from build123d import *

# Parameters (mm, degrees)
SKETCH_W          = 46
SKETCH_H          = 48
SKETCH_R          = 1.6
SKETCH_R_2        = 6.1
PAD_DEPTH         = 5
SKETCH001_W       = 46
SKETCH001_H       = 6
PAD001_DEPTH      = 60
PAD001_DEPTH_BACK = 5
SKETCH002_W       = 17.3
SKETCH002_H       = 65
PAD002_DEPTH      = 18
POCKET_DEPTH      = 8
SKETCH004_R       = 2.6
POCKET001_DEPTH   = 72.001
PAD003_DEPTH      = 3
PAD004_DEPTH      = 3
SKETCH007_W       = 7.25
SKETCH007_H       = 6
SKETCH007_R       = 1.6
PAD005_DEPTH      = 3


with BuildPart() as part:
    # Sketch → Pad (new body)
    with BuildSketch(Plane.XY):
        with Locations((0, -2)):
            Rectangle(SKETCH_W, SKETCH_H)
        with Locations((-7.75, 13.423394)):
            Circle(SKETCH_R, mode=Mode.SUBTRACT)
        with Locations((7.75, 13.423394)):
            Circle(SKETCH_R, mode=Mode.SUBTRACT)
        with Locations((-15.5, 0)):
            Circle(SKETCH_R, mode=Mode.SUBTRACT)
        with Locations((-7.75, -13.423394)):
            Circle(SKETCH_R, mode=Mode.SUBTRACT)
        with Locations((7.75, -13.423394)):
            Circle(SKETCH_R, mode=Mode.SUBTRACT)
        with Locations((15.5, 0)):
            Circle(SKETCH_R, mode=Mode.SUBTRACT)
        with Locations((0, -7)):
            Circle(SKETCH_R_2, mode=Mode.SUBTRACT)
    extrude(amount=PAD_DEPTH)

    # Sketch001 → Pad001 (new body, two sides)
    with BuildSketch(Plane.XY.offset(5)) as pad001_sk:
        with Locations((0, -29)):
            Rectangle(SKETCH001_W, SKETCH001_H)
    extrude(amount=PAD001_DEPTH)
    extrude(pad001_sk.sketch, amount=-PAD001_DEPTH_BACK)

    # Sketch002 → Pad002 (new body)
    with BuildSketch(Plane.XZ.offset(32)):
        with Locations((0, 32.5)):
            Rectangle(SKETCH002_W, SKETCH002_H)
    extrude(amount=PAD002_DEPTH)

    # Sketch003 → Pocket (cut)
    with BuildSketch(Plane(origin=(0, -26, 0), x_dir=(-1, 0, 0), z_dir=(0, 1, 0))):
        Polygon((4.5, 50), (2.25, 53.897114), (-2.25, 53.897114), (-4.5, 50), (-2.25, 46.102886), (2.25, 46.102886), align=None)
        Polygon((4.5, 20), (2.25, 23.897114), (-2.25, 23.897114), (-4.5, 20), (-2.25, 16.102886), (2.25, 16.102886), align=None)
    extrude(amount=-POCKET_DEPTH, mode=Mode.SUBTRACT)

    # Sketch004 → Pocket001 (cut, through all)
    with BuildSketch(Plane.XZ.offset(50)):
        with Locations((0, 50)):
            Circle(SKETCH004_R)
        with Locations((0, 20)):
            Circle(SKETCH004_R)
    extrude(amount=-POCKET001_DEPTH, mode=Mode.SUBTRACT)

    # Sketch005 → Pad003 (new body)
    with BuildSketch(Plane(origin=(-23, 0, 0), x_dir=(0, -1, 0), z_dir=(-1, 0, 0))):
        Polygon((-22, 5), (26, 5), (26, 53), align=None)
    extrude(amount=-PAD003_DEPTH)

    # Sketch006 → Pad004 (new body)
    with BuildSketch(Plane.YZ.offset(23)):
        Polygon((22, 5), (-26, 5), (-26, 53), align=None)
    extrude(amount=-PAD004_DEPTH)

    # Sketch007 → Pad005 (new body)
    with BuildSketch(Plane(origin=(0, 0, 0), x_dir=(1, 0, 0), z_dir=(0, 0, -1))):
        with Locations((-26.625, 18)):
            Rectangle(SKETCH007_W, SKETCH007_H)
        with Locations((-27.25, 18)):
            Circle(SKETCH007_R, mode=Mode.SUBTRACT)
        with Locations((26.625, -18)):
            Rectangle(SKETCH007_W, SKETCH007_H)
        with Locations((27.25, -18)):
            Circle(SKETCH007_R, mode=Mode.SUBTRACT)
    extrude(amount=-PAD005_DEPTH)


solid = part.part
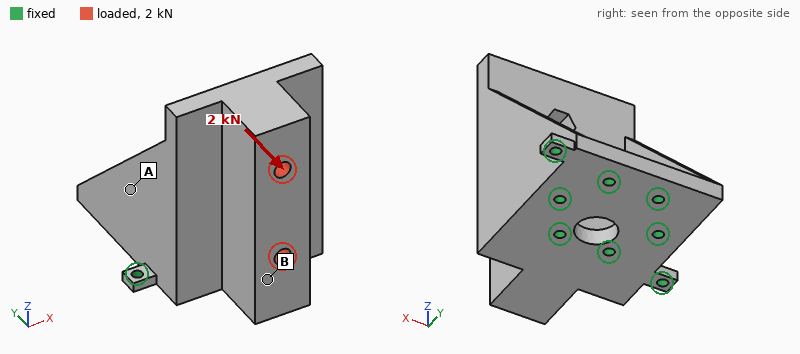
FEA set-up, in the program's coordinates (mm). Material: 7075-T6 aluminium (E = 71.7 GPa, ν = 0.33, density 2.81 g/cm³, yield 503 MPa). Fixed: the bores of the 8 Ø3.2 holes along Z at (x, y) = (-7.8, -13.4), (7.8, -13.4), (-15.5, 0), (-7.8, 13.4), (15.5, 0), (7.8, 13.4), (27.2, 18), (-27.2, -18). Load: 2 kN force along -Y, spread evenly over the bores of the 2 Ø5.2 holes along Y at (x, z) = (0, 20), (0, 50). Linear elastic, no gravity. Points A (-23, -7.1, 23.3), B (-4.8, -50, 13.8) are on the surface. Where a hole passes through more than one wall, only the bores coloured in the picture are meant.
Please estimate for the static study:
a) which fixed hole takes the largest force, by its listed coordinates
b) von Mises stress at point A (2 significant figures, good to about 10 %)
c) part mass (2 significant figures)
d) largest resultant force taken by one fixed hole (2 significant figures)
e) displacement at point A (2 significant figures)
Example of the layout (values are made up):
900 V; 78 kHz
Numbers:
(-15.5, 0); 19 MPa; 150 g; 1.2 kN; 0.042 mm
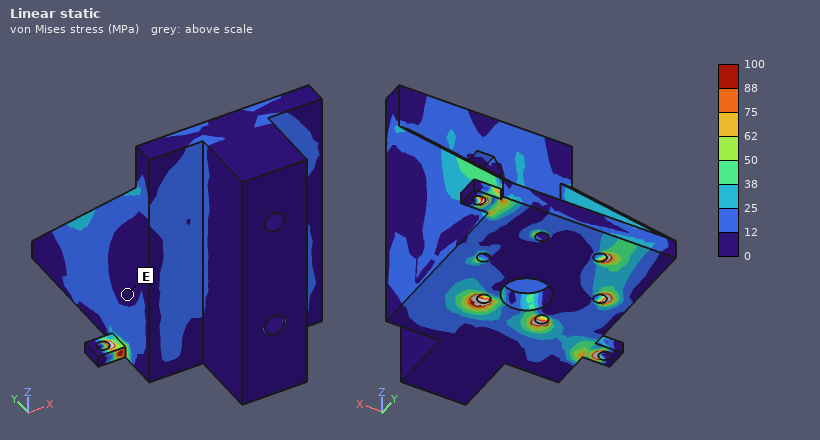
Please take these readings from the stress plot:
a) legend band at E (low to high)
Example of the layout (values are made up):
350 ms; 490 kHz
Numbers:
0 to 12 MPa
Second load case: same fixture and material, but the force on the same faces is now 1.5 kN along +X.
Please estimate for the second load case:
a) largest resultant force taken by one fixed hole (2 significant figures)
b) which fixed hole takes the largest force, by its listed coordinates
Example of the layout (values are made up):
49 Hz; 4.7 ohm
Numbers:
1.2 kN; (7.8, -13.4)
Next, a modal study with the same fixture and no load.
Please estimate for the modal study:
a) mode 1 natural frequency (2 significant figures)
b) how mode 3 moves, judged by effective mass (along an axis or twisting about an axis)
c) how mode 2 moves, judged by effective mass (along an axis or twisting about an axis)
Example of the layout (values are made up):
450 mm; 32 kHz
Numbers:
1800 Hz; along Z; along X
